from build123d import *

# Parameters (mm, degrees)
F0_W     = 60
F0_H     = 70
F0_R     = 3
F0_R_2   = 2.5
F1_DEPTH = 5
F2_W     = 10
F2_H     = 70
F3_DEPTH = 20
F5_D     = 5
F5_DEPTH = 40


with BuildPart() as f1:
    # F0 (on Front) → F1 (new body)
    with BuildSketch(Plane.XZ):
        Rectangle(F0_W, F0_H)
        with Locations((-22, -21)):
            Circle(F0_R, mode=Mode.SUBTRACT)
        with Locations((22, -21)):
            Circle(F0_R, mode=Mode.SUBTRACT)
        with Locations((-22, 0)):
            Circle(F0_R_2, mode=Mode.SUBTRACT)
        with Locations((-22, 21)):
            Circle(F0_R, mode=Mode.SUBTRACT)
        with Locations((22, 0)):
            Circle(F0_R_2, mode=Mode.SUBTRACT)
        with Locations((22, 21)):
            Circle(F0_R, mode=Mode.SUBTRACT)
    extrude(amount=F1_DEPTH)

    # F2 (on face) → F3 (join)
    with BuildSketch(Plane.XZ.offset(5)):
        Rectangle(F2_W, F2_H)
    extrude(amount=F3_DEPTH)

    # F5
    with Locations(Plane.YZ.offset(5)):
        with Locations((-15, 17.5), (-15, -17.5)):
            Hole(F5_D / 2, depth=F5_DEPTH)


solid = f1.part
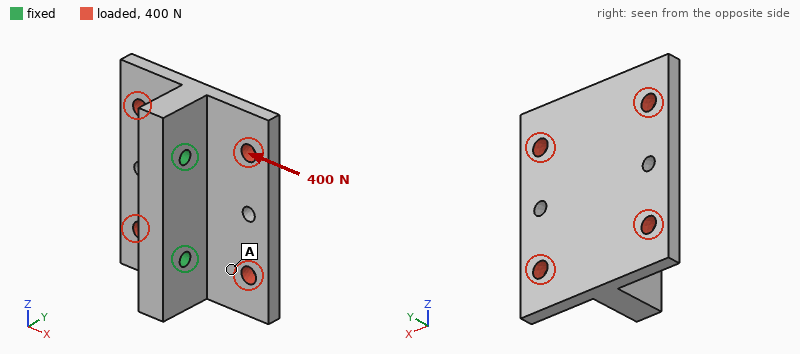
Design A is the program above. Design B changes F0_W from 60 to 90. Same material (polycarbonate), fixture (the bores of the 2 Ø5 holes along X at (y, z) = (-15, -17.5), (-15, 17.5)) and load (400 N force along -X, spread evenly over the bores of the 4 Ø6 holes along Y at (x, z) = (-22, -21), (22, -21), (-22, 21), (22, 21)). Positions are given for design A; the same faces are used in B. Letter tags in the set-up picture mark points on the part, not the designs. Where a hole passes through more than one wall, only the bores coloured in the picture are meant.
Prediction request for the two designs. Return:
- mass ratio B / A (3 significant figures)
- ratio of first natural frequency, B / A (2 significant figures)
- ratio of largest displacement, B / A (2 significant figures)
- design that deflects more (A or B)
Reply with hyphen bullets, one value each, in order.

- 1.31
- 0.46
- 1.4
- B
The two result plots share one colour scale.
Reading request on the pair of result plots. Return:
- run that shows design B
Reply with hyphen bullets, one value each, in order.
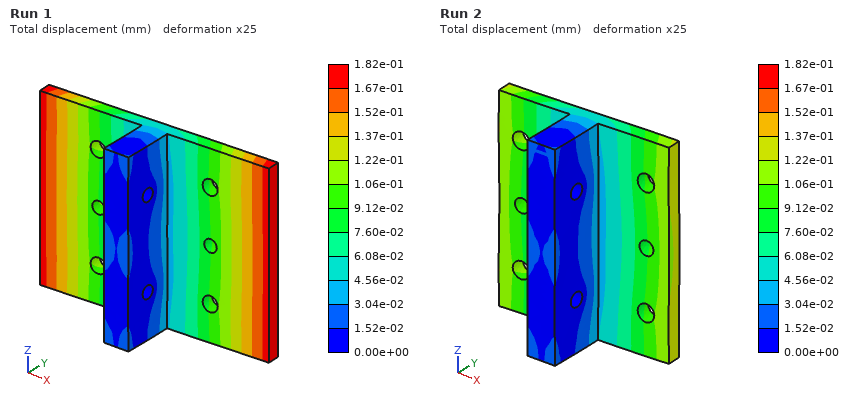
- Run 1
